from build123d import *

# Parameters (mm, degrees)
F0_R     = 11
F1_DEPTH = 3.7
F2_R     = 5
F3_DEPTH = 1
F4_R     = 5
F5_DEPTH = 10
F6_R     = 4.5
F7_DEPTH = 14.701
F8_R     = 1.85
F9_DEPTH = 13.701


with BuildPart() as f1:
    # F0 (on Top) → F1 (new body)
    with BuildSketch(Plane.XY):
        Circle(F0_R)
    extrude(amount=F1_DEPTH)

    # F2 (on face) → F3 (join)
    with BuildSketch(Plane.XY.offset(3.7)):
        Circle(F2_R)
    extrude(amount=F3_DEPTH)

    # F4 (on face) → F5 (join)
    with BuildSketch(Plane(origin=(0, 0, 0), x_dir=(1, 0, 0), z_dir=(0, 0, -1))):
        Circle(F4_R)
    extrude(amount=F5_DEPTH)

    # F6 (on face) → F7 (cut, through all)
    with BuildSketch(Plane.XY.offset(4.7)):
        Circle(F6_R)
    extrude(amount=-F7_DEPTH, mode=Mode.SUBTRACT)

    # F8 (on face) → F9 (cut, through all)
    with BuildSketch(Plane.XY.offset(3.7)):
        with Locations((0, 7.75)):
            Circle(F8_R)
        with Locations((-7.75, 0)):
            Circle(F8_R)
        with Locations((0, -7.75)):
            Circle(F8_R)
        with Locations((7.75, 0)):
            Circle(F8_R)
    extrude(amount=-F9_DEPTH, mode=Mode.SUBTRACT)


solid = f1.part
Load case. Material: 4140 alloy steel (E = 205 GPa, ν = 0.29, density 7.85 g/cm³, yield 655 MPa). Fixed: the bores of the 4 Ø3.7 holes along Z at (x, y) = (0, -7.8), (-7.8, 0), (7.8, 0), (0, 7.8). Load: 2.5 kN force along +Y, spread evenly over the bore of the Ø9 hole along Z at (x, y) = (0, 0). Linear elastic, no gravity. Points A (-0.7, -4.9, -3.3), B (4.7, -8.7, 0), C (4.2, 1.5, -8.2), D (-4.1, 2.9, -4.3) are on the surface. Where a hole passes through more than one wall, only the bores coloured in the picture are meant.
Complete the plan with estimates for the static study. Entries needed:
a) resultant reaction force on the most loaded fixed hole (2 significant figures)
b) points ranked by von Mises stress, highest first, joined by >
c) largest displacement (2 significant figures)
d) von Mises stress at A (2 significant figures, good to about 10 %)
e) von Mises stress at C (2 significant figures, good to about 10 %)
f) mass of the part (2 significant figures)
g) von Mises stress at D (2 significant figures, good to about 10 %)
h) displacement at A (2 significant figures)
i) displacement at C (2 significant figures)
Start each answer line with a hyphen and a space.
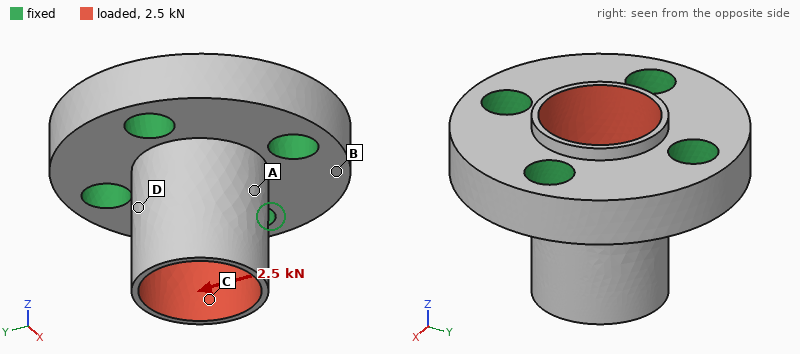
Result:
- 1.0 kN
- D > A > C > B
- 27 µm
- 130 MPa
- 73 MPa
- 9.2 g
- 190 MPa
- 14 µm
- 23 µm
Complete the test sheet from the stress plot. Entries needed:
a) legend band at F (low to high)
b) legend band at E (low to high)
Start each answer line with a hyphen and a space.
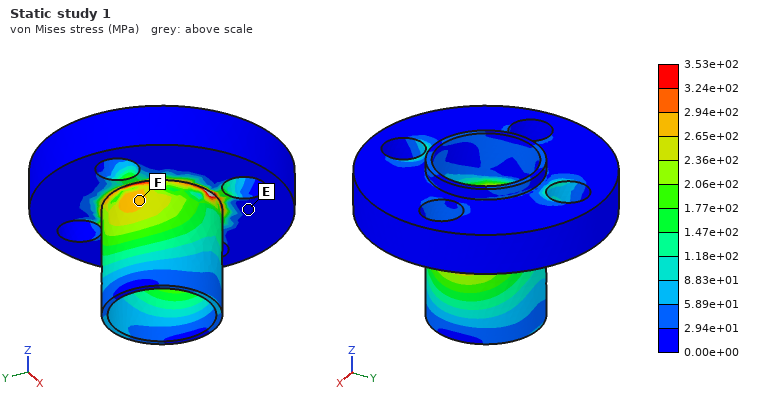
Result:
- 2.65e+02 to 2.94e+02 MPa
- 0.00e+00 to 2.94e+01 MPa
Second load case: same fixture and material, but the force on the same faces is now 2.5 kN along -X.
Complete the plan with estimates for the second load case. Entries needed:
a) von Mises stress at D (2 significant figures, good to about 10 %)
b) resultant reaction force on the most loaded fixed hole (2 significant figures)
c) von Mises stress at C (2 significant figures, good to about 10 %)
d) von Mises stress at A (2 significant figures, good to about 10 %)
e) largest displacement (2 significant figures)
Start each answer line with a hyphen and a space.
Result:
- 150 MPa
- 1.0 kN
- 68 MPa
- 250 MPa
- 27 µm
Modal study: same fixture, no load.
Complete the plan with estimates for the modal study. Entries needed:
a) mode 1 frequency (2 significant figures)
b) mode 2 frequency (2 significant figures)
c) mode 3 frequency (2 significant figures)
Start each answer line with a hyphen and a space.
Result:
- 26 kHz
- 27 kHz
- 43 kHz
